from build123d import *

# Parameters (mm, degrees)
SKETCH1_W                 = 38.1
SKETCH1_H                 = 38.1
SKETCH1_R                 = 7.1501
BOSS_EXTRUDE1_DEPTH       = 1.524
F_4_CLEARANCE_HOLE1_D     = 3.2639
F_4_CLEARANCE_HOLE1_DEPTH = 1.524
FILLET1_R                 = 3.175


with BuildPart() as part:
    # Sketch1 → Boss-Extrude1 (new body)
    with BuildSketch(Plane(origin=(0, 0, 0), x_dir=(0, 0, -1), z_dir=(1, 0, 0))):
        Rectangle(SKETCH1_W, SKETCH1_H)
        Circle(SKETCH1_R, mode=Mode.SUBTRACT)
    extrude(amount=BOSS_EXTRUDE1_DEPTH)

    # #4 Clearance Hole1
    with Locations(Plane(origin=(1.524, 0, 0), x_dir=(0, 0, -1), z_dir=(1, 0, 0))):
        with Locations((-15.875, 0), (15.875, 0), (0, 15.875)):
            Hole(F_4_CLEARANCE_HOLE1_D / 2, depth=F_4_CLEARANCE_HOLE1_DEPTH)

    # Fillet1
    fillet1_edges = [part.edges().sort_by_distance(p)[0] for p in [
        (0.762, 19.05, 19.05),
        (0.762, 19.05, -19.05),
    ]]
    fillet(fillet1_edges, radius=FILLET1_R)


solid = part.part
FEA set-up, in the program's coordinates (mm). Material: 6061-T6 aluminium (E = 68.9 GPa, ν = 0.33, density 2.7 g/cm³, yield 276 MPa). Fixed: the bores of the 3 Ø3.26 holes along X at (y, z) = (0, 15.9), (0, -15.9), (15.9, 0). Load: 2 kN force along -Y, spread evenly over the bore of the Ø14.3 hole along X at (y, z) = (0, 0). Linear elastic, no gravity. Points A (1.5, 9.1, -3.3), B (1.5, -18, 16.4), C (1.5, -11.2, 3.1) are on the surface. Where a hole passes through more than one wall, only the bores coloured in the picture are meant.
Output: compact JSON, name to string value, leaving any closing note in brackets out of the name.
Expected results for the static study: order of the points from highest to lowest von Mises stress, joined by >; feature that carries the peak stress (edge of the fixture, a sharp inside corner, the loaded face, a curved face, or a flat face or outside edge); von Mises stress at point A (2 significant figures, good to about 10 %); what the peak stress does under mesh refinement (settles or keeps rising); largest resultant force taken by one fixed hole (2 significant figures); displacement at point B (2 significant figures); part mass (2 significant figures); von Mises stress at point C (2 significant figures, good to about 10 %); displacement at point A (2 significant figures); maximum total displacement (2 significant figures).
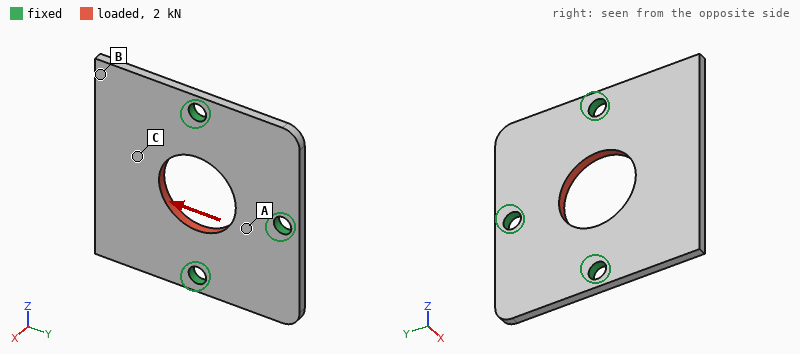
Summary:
{"order of the points from highest to lowest von Mises stress, joined by >": "A > C > B", "feature that carries the peak stress": "edge of the fixture", "von Mises stress at point A": "41 MPa", "what the peak stress does under mesh refinement": "keeps rising", "largest resultant force taken by one fixed hole": "700 N", "displacement at point B": "5.3 µm", "part mass": "5.2 g", "von Mises stress at point C": "28 MPa", "displacement at point A": "4.7 µm", "maximum total displacement": "14 µm"}
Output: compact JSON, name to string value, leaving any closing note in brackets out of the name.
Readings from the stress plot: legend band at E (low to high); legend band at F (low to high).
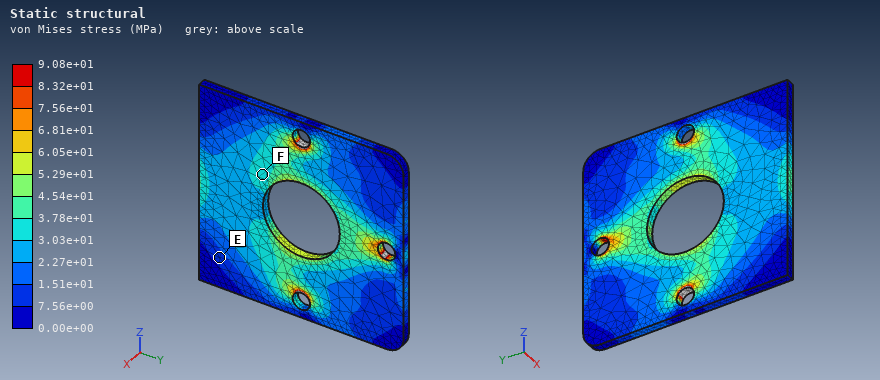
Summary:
{"legend band at E": "7.56e+00 to 1.51e+01 MPa", "legend band at F": "3.03e+01 to 3.78e+01 MPa"}
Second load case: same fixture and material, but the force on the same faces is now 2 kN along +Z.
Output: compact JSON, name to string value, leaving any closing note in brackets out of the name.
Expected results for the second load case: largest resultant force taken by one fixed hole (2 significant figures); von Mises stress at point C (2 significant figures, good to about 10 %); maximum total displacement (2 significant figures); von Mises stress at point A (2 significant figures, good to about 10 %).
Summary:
{"largest resultant force taken by one fixed hole": "810 N", "von Mises stress at point C": "10 MPa", "maximum total displacement": "13 µm", "von Mises stress at point A": "22 MPa"}
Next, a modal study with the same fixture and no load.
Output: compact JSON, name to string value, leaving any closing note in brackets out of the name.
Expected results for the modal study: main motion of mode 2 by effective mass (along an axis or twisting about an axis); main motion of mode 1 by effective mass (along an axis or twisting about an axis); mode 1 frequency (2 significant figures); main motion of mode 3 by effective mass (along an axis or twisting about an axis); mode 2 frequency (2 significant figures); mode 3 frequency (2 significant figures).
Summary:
{"main motion of mode 2 by effective mass": "twisting about Y", "main motion of mode 1 by effective mass": "along X", "mode 1 frequency": "2800 Hz", "main motion of mode 3 by effective mass": "along X", "mode 2 frequency": "5500 Hz", "mode 3 frequency": "7600 Hz"}
